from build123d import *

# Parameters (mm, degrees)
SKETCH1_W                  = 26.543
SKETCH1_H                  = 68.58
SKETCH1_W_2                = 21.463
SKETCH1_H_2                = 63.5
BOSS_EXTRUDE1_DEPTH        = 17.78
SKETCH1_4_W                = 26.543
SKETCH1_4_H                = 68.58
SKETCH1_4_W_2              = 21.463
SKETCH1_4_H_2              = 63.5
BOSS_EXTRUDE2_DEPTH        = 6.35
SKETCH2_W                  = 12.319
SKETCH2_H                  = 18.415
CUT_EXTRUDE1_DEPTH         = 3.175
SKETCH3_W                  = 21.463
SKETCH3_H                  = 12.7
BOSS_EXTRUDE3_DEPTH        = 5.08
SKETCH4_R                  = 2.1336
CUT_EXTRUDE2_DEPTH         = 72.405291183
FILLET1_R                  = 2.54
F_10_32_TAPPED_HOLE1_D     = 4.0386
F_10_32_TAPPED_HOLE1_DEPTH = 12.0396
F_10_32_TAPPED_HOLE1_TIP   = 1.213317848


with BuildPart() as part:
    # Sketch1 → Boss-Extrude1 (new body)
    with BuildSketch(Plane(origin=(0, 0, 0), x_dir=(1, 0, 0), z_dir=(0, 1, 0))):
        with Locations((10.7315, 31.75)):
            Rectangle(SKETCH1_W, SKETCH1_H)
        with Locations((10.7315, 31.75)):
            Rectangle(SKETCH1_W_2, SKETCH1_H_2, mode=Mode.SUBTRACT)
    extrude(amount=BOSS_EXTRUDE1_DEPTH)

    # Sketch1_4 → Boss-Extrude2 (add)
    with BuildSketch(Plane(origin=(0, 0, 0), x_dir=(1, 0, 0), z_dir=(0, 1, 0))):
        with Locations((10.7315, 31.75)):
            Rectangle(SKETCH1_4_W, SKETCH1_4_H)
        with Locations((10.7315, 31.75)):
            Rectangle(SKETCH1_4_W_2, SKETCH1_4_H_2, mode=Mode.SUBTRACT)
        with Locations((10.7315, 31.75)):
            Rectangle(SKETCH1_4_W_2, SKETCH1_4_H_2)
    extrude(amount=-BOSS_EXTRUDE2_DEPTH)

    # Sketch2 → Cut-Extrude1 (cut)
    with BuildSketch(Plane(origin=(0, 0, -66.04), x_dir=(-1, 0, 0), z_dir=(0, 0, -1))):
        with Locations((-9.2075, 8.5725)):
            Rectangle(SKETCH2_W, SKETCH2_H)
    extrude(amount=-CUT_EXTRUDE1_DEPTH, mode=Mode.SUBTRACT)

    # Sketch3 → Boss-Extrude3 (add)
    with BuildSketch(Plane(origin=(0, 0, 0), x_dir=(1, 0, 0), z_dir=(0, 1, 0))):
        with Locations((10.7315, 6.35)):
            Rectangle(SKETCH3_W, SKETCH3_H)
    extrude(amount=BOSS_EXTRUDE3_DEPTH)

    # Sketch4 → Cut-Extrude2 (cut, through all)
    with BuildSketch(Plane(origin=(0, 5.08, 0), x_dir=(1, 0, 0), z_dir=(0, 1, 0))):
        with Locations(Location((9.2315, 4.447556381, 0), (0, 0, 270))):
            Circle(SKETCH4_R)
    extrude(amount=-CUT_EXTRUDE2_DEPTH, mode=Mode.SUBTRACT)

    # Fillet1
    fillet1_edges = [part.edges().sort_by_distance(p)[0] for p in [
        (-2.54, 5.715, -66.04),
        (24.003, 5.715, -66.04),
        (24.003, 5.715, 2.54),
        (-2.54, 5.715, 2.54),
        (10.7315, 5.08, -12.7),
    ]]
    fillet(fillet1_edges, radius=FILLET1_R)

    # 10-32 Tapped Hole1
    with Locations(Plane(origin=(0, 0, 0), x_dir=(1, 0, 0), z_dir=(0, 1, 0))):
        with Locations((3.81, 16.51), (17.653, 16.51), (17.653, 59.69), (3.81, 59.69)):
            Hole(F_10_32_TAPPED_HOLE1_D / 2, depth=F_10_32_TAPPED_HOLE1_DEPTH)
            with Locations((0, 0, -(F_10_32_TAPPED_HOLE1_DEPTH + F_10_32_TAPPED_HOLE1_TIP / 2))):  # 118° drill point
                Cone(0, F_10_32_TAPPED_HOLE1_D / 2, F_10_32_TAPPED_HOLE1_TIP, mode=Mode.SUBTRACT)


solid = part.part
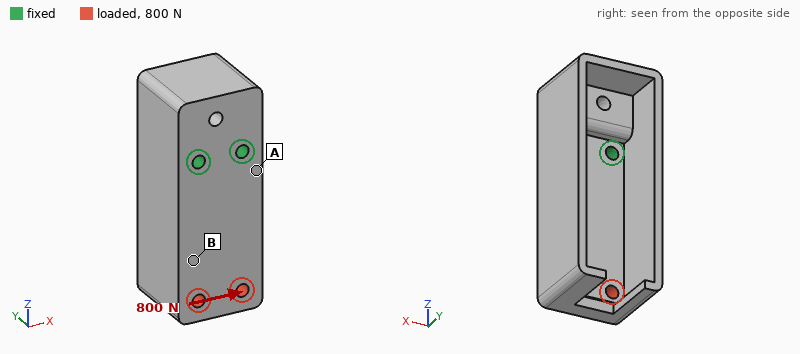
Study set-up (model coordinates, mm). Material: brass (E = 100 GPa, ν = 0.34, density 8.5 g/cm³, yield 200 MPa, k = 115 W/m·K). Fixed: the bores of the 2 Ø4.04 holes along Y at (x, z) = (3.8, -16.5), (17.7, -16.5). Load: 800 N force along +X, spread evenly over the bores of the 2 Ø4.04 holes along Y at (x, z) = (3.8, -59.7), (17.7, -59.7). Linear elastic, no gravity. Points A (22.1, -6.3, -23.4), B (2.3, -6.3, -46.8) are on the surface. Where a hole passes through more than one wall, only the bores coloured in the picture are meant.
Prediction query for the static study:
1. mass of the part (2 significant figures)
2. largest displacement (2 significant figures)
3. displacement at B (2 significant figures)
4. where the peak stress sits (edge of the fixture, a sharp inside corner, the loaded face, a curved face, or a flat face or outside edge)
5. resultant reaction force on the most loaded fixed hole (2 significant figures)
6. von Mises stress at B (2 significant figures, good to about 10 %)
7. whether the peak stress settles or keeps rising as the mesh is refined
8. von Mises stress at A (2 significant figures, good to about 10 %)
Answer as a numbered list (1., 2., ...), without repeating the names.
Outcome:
1. 170 g
2. 40 µm
3. 16 µm
4. edge of the fixture
5. 2.1 kN
6. 7.3 MPa
7. keeps rising
8. 25 MPa
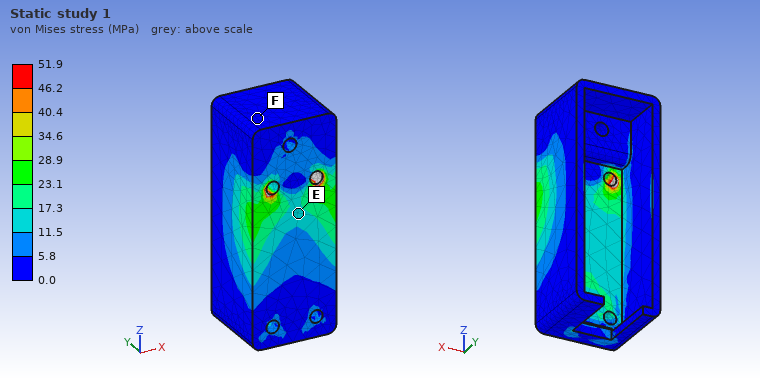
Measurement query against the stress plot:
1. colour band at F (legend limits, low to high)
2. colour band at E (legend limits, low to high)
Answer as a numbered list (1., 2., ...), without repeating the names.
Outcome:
1. 0.0 to 5.8 MPa
2. 11.5 to 17.3 MPa
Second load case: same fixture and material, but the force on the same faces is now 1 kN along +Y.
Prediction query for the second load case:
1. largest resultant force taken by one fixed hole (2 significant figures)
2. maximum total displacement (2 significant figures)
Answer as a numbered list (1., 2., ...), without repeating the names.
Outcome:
1. 510 N
2. 0.15 mm
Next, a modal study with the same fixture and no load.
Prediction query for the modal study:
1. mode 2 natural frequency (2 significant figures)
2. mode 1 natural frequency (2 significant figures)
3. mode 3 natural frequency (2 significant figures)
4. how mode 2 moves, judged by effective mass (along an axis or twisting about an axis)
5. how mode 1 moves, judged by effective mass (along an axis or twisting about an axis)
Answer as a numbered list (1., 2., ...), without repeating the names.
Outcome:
1. 2700 Hz
2. 2000 Hz
3. 4400 Hz
4. along X
5. along Y
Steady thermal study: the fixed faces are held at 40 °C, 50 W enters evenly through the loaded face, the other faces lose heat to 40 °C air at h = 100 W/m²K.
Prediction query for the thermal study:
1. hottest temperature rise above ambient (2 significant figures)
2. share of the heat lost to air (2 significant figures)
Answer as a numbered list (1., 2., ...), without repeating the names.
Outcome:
1. 61 K
2. 44 %
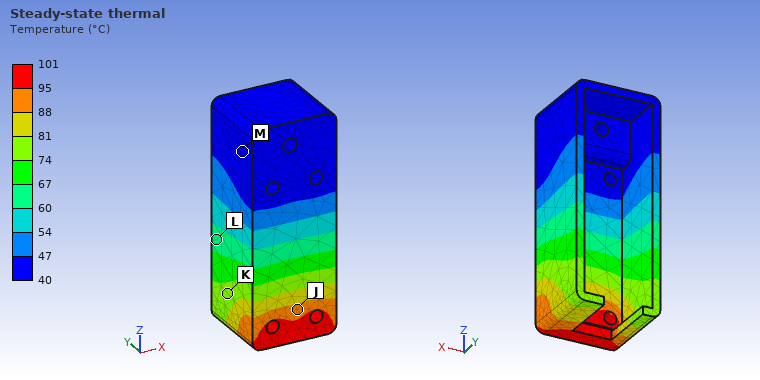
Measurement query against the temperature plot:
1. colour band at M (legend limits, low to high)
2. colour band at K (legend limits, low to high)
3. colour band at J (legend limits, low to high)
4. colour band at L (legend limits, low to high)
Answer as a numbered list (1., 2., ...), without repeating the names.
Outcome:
1. 40 to 47 °C
2. 74 to 81 °C
3. 88 to 95 °C
4. 60 to 67 °C
